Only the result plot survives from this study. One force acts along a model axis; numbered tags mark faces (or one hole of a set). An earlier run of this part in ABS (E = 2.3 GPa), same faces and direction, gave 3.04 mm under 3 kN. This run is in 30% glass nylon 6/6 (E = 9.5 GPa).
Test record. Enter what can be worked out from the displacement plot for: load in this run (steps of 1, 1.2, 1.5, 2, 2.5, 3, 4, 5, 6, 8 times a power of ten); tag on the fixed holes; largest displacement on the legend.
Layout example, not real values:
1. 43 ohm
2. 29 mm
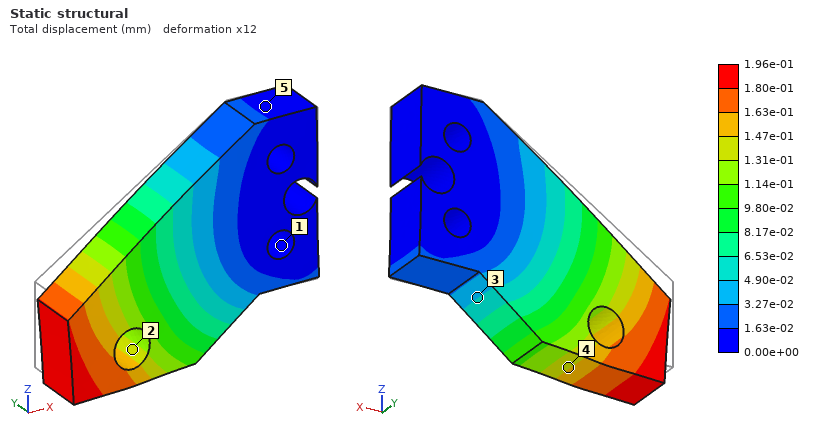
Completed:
1. 800 N
2. 1
3. 1.96e-01 mm
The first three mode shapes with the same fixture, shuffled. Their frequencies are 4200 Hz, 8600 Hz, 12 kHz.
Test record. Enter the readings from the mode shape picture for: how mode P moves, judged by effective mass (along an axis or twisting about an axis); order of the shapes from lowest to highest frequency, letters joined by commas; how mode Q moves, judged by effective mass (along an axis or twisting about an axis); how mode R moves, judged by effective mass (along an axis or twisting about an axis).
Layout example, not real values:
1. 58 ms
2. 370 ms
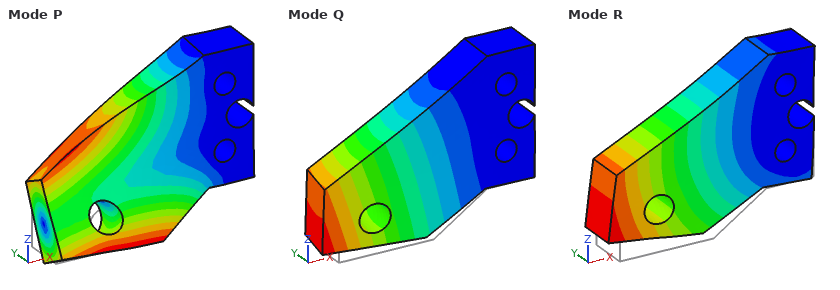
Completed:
1. twisting about X
2. Q, R, P
3. along Y
4. along Z
